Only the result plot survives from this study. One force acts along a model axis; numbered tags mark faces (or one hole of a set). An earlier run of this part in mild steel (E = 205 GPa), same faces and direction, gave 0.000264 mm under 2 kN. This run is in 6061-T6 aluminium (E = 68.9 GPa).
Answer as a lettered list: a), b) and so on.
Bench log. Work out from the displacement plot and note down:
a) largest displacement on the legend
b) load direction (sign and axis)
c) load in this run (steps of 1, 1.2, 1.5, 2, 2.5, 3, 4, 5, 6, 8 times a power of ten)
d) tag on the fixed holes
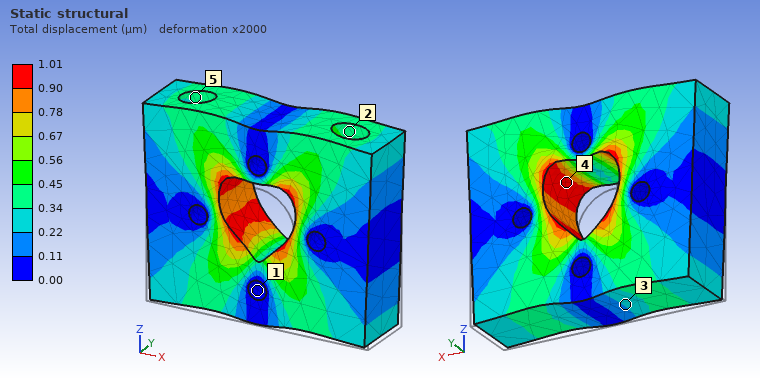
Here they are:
a) 1.01 µm
b) +Z
c) 2.5 kN
d) 1
